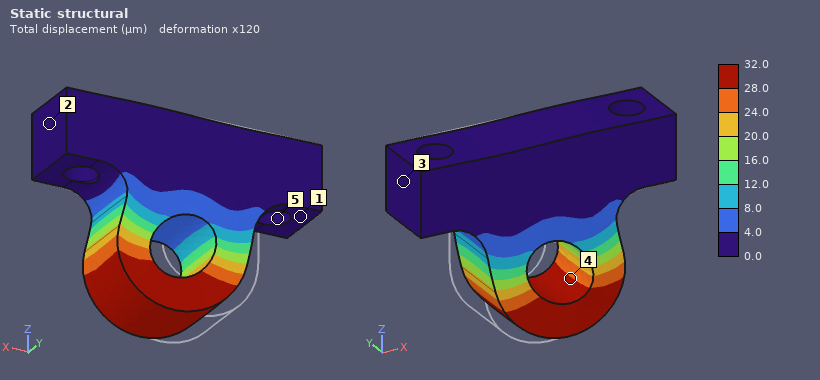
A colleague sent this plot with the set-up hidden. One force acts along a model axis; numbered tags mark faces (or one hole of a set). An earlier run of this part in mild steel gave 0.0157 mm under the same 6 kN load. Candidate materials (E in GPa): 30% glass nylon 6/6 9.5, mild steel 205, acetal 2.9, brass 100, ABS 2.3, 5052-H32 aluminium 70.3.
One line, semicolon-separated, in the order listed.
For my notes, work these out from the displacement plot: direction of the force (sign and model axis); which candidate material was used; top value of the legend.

+X; brass; 32.0 µm
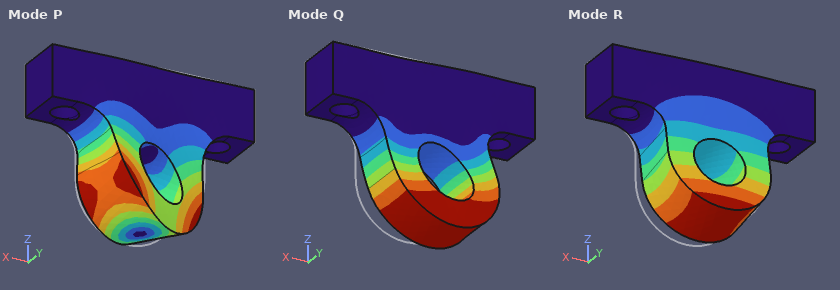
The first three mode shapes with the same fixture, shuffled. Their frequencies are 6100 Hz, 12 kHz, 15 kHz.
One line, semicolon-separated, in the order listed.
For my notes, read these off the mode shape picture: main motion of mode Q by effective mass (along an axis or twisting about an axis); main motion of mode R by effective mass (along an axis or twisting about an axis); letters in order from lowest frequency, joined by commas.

along X; along Y; R, Q, P
